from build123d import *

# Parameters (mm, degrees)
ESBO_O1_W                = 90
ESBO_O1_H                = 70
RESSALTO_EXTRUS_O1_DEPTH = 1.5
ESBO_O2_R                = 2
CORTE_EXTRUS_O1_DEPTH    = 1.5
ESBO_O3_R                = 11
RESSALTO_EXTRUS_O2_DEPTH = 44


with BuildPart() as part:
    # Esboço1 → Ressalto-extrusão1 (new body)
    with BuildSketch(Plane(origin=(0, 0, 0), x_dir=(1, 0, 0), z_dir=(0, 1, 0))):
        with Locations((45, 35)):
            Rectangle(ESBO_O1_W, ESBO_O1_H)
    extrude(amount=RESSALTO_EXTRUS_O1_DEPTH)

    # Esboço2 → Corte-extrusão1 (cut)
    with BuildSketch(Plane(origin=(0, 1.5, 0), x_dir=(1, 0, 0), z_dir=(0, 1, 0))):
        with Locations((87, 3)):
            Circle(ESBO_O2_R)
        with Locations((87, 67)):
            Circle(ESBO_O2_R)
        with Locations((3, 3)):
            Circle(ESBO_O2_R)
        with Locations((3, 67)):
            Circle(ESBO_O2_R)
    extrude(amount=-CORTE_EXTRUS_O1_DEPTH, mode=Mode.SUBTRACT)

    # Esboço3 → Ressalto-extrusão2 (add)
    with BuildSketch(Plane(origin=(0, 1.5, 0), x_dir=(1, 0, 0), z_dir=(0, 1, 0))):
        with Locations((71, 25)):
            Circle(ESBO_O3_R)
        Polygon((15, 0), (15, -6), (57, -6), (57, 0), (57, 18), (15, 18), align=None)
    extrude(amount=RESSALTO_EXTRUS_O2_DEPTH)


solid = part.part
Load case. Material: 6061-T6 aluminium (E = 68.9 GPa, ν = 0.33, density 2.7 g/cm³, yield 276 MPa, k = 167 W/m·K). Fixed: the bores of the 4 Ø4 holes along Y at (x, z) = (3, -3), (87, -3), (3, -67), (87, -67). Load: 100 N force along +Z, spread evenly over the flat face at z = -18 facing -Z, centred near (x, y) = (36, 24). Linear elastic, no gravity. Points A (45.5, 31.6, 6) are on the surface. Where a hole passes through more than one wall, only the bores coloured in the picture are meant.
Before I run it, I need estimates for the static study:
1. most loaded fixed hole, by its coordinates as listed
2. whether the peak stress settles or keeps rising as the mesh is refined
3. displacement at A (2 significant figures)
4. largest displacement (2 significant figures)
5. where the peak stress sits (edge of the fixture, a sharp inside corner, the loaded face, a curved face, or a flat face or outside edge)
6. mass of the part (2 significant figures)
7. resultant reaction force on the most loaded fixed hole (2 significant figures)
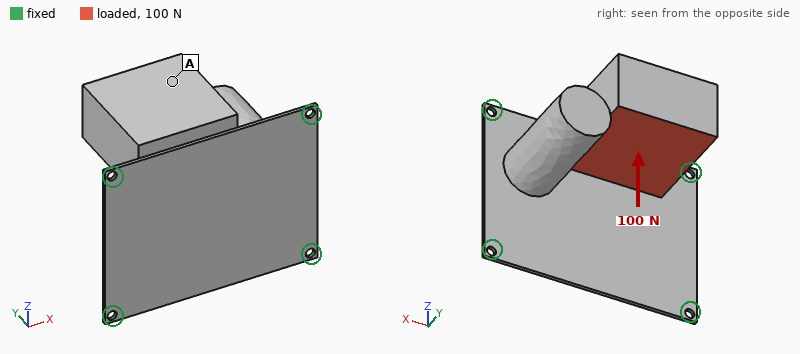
(3, -3)
keeps rising
0.28 mm
0.38 mm
edge of the fixture
190 g
43 N
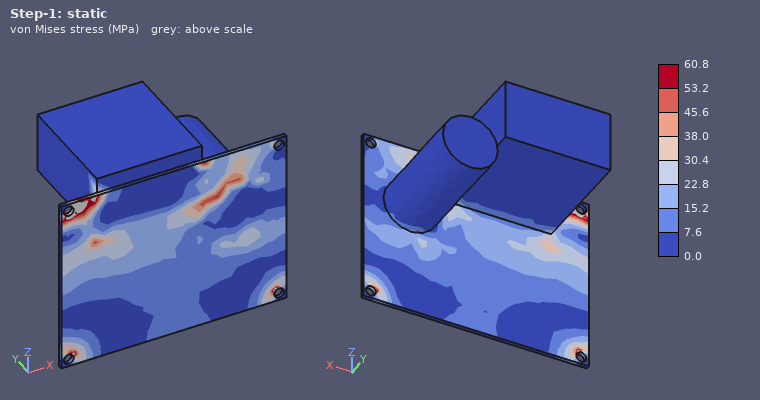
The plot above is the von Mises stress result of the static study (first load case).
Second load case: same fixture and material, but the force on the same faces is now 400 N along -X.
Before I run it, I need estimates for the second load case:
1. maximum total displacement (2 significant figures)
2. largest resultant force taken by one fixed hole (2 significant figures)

0.47 mm
220 N
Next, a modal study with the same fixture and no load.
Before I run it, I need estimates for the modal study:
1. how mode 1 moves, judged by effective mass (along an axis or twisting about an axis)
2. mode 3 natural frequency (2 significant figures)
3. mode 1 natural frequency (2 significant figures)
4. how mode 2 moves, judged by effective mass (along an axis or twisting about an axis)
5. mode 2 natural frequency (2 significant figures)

along Z
560 Hz
270 Hz
along Y
330 Hz
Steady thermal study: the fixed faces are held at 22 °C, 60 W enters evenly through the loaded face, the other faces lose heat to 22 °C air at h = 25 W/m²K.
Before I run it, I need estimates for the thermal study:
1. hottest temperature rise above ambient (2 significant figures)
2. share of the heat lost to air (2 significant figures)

74 K
36 %
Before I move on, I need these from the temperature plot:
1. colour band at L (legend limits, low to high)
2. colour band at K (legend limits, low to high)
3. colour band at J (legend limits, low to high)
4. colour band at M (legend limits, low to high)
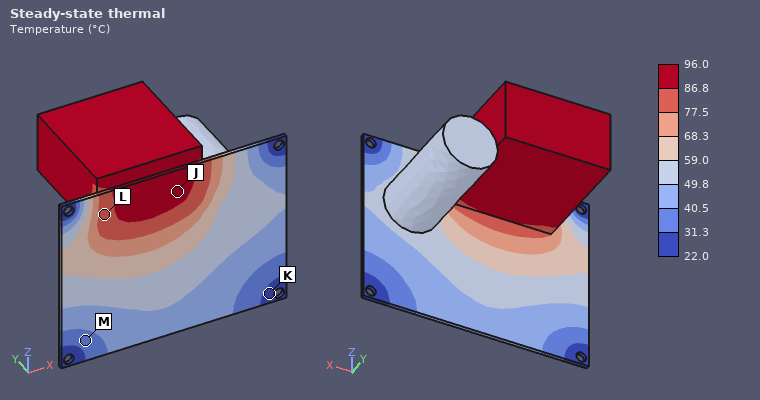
77.5 to 86.8 °C
22.0 to 31.3 °C
86.8 to 96.0 °C
31.3 to 40.5 °C
